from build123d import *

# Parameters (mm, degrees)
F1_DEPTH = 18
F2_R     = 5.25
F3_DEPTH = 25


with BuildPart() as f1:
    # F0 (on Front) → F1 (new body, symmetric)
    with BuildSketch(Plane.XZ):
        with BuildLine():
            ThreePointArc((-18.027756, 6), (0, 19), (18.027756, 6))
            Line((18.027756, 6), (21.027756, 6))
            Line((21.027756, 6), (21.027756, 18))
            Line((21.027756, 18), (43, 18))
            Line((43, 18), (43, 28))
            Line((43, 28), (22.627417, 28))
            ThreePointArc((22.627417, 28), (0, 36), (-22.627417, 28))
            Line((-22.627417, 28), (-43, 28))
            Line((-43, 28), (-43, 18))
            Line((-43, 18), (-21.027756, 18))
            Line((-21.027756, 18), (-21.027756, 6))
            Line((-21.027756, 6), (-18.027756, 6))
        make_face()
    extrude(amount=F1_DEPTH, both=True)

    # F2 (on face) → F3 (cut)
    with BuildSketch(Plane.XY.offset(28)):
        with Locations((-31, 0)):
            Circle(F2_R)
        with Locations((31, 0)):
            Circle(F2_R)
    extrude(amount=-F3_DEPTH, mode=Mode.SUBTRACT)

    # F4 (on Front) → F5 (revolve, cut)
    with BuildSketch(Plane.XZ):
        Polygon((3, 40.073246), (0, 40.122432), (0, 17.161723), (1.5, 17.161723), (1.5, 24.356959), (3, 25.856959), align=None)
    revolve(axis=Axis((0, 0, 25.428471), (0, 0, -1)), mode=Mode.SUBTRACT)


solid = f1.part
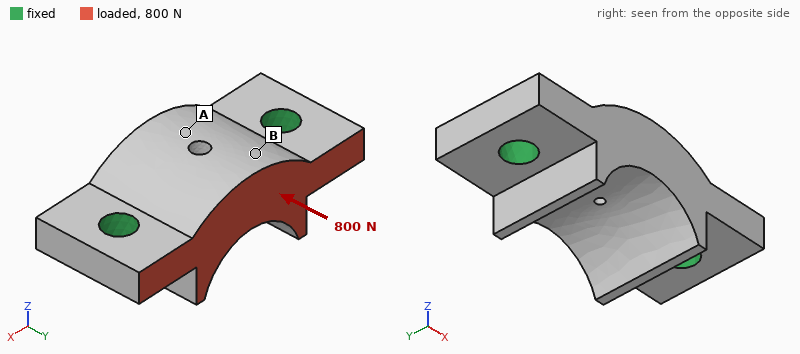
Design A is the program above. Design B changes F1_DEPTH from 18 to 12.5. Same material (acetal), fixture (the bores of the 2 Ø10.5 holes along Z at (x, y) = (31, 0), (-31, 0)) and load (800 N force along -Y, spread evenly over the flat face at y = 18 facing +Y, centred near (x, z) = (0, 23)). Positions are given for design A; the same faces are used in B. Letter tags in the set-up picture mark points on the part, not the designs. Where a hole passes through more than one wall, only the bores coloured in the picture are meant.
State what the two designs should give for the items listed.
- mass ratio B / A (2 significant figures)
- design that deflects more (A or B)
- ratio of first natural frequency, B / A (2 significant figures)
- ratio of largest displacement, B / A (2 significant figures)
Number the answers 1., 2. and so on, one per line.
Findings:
1. 0.68
2. B
3. 1.2
4. 1.4
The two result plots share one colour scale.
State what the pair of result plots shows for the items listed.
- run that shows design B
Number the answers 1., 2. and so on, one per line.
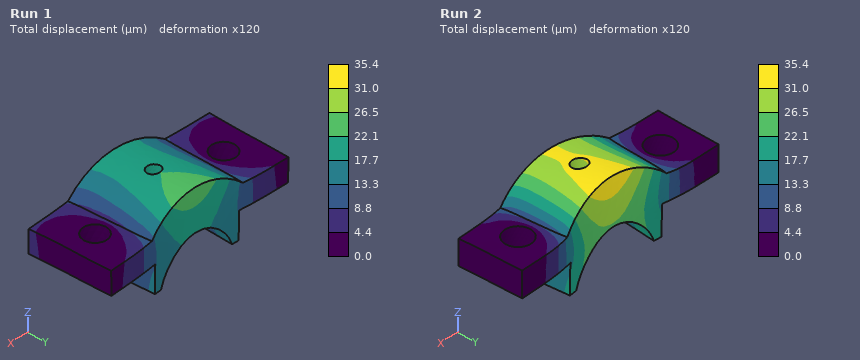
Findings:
1. Run 2
